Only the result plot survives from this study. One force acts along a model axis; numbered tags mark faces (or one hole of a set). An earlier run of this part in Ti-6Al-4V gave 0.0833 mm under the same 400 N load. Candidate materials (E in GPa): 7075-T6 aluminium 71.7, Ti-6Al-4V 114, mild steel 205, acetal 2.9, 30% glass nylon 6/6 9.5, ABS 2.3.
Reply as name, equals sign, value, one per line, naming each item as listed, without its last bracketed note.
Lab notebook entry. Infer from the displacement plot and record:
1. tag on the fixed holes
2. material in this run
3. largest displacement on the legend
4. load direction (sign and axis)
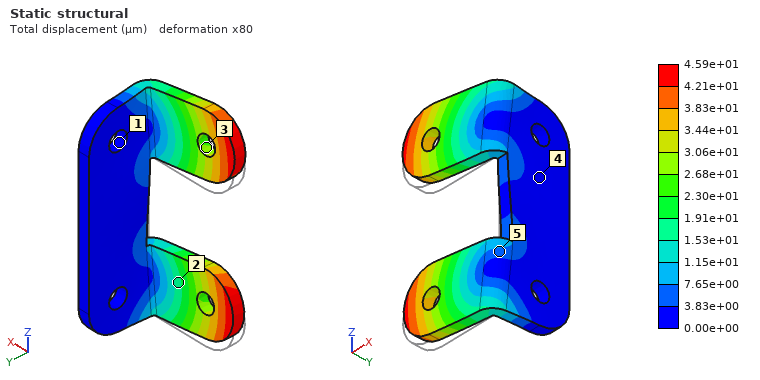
tag on the fixed holes = 1
material in this run = mild steel
largest displacement on the legend = 4.59e+01 µm
load direction = +Z
